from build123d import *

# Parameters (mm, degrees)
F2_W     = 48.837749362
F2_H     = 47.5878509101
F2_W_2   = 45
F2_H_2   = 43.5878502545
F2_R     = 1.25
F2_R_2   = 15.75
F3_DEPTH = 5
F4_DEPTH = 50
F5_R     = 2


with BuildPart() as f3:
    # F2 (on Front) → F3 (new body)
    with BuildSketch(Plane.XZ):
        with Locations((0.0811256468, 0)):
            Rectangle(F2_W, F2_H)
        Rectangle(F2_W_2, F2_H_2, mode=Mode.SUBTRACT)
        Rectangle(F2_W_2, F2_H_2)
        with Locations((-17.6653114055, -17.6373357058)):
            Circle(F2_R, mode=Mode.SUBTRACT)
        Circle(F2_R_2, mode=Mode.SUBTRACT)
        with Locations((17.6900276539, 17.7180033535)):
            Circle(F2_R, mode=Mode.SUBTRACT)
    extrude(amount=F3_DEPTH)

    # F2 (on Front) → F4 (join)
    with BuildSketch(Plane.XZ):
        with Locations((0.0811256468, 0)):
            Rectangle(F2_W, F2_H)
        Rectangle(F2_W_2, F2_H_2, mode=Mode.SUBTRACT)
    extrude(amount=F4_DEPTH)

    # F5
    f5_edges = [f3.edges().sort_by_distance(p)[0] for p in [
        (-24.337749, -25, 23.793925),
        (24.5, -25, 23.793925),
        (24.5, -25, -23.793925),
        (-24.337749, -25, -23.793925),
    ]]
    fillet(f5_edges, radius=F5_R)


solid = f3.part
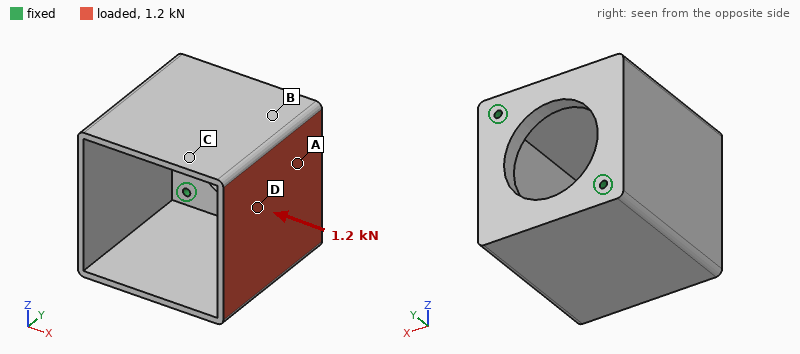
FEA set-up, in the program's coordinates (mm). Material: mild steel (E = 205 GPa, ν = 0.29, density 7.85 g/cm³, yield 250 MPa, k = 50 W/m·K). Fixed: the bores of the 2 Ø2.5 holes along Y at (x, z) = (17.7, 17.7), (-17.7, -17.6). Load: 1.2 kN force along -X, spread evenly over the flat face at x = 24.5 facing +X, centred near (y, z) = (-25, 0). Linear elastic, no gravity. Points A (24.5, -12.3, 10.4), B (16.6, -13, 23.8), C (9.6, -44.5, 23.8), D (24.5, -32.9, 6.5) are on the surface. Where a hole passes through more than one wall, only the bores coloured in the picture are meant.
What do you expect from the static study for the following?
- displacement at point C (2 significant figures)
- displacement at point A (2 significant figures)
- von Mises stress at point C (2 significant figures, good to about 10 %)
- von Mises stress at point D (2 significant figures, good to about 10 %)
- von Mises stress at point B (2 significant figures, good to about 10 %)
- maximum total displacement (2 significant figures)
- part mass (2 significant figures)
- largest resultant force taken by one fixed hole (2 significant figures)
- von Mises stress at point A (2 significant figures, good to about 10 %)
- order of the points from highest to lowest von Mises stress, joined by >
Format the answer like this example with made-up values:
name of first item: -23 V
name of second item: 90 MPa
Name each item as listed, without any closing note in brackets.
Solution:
displacement at point C: 0.075 mm
displacement at point A: 0.026 mm
von Mises stress at point C: 36 MPa
von Mises stress at point D: 70 MPa
von Mises stress at point B: 18 MPa
maximum total displacement: 0.15 mm
part mass: 190 g
largest resultant force taken by one fixed hole: 710 N
von Mises stress at point A: 51 MPa
order of the points from highest to lowest von Mises stress, joined by >: D > A > C > B
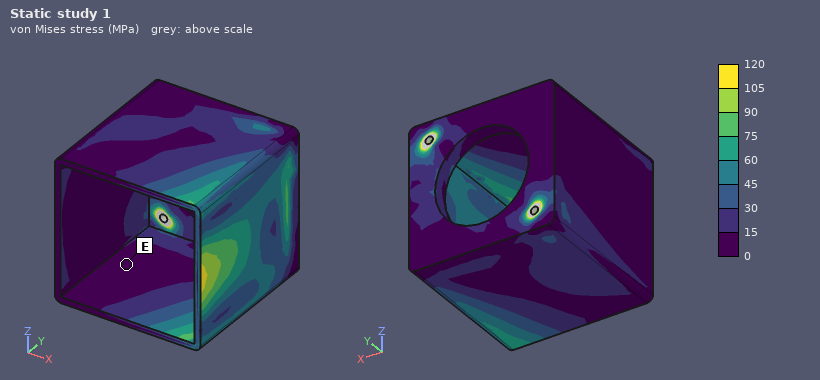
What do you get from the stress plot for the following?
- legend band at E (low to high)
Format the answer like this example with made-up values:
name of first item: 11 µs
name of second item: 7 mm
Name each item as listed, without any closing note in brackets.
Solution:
legend band at E: 0 to 15 MPa
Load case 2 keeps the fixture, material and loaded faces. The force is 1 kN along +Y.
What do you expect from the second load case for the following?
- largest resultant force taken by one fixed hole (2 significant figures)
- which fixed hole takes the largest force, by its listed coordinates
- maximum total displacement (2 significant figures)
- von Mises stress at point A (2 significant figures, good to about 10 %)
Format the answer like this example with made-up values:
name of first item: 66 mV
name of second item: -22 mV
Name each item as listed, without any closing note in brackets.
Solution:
largest resultant force taken by one fixed hole: 820 N
which fixed hole takes the largest force, by its listed coordinates: (17.7, 17.7)
maximum total displacement: 92 µm
von Mises stress at point A: 24 MPa
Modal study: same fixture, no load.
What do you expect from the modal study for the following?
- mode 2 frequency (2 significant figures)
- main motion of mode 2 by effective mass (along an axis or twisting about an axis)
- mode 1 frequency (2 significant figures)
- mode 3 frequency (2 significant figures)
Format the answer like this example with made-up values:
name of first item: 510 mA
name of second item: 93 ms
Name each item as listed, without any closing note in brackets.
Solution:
mode 2 frequency: 2000 Hz
main motion of mode 2 by effective mass: along Y
mode 1 frequency: 1600 Hz
mode 3 frequency: 2800 Hz
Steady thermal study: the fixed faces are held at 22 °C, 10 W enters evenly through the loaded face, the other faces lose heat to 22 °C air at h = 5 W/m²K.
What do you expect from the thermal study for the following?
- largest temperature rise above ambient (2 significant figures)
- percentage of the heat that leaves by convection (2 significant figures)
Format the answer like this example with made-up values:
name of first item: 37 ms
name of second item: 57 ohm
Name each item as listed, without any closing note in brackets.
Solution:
largest temperature rise above ambient: 35 K
percentage of the heat that leaves by convection: 13 %
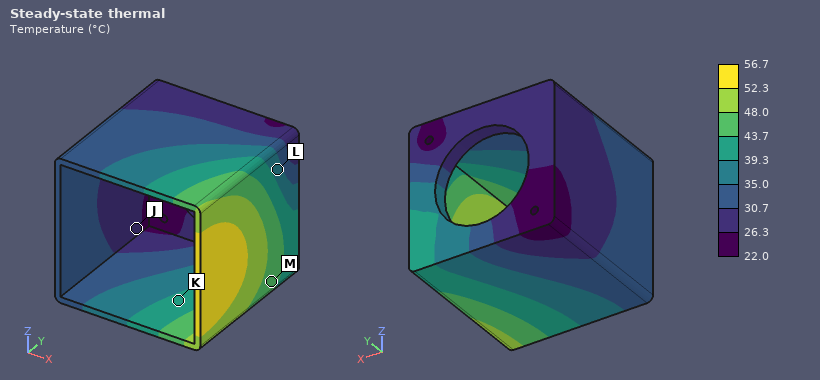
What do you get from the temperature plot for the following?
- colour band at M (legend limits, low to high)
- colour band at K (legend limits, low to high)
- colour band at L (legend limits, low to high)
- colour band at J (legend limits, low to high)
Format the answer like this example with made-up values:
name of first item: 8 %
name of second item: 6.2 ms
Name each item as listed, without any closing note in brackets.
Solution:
colour band at M: 43.7 to 48.0 °C
colour band at K: 39.3 to 43.7 °C
colour band at L: 35.0 to 39.3 °C
colour band at J: 26.3 to 30.7 °C
